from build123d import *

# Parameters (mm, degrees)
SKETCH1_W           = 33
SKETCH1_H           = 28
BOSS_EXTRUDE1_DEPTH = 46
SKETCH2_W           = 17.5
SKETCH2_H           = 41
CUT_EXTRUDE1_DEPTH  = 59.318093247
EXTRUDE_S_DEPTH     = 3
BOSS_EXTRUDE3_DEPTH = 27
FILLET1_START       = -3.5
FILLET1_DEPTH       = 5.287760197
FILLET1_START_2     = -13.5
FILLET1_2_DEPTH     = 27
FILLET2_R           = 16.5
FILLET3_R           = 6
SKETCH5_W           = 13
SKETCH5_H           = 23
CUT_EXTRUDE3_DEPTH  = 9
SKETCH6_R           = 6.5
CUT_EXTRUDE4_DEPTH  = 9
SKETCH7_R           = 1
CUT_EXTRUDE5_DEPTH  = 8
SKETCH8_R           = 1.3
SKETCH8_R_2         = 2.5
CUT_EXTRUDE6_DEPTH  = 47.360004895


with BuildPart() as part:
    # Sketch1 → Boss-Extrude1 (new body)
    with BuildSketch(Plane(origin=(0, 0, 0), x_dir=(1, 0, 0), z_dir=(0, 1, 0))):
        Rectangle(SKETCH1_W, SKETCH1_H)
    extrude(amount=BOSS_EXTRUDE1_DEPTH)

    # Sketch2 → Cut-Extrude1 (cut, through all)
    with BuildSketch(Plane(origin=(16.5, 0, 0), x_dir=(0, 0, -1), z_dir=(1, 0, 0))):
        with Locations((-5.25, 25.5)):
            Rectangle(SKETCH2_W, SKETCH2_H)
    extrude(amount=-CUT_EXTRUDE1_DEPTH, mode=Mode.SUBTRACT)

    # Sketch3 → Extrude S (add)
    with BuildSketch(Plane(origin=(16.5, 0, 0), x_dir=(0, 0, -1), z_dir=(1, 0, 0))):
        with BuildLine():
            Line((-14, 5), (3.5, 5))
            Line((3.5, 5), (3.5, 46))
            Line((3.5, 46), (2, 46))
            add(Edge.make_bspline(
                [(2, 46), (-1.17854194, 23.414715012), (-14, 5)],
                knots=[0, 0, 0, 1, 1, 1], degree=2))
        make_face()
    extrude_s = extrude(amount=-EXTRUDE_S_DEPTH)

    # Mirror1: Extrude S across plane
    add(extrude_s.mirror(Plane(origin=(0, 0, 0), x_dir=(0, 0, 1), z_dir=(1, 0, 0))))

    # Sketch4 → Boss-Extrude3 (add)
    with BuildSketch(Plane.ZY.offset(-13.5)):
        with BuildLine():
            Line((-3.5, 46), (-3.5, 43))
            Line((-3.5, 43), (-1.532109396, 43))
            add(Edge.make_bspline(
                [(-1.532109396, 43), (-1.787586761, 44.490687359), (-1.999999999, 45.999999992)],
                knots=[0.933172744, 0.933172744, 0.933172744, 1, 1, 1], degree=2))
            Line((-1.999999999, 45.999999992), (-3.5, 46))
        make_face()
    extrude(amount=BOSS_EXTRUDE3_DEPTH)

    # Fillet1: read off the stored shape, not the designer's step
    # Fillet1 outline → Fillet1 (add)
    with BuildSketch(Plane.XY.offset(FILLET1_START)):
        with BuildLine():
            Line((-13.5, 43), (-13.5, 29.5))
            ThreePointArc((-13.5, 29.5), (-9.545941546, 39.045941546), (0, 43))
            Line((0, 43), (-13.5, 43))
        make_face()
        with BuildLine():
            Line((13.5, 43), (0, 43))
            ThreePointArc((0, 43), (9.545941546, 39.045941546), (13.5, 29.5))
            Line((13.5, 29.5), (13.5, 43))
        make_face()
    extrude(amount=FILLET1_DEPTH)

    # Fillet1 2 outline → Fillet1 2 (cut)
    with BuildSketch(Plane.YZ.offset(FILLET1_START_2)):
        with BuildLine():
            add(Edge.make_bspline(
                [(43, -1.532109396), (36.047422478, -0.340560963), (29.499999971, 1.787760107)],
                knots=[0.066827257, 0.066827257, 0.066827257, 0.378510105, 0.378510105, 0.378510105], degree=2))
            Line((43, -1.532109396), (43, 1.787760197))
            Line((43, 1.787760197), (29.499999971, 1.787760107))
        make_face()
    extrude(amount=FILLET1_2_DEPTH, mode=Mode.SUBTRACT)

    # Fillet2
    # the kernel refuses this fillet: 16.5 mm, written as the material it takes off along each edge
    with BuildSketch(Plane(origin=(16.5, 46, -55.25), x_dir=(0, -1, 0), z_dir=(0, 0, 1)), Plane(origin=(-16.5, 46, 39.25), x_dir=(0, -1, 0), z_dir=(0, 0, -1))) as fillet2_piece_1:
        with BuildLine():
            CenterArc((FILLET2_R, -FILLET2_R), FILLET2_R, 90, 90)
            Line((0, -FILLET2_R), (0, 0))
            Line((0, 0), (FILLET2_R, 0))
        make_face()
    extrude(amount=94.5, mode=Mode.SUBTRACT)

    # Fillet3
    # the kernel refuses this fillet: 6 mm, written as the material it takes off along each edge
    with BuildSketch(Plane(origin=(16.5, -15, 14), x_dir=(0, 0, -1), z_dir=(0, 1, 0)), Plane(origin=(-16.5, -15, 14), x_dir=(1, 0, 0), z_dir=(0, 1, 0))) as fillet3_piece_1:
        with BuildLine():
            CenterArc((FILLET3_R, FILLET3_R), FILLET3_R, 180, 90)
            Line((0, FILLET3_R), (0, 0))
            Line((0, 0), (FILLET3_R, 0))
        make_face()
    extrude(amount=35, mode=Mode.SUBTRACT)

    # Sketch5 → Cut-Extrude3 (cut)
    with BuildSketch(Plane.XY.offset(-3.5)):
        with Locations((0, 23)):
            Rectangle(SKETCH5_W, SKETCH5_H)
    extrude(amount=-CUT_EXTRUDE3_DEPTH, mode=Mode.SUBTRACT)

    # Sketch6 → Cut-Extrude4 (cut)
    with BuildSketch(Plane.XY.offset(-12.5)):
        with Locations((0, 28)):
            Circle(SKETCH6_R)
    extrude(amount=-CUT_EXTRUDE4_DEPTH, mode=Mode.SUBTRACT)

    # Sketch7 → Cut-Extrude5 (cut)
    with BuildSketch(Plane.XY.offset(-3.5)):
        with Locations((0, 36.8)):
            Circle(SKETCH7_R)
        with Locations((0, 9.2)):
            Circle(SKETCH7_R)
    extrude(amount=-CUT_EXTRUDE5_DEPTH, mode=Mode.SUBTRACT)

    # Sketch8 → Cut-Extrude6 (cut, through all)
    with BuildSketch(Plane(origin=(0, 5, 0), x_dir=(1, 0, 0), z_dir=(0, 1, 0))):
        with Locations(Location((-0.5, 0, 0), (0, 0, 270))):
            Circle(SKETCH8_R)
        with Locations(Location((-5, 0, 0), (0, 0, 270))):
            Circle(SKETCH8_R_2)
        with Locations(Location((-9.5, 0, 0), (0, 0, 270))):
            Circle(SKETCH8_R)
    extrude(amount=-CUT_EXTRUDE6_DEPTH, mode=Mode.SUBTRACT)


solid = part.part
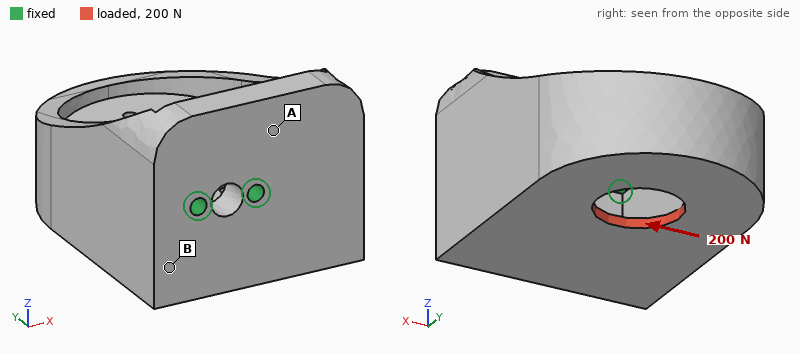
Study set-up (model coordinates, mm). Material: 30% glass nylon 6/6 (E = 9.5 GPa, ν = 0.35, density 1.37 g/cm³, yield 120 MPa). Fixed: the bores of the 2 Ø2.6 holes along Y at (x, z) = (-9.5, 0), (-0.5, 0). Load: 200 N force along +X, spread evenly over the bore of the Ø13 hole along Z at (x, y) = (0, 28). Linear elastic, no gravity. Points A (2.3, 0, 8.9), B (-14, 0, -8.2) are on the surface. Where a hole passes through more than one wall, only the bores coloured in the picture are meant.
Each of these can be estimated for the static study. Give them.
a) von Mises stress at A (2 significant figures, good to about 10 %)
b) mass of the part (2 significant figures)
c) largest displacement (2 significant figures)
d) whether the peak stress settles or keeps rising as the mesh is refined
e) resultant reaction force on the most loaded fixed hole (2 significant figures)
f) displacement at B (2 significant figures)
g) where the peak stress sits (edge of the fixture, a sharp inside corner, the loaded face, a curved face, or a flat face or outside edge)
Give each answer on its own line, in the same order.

6.1 MPa
22 g
0.16 mm
keeps rising
430 N
0.025 mm
edge of the fixture
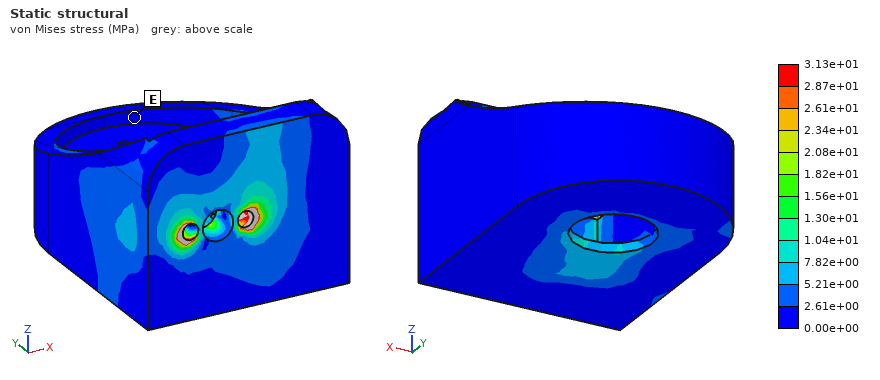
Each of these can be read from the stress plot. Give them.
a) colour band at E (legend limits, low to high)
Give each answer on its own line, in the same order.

0.00e+00 to 2.61e+00 MPa
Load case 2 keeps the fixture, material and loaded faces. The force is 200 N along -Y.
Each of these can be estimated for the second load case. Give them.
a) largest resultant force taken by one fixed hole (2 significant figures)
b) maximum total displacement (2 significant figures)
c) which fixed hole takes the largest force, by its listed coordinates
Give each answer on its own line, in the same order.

160 N
0.17 mm
(-0.5, 0)
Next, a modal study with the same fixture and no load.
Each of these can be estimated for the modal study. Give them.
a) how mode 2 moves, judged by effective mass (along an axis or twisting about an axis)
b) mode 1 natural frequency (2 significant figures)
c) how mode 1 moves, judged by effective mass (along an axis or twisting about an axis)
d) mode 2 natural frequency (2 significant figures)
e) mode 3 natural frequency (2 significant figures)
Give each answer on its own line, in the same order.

along X
1200 Hz
along Z
1700 Hz
3800 Hz
